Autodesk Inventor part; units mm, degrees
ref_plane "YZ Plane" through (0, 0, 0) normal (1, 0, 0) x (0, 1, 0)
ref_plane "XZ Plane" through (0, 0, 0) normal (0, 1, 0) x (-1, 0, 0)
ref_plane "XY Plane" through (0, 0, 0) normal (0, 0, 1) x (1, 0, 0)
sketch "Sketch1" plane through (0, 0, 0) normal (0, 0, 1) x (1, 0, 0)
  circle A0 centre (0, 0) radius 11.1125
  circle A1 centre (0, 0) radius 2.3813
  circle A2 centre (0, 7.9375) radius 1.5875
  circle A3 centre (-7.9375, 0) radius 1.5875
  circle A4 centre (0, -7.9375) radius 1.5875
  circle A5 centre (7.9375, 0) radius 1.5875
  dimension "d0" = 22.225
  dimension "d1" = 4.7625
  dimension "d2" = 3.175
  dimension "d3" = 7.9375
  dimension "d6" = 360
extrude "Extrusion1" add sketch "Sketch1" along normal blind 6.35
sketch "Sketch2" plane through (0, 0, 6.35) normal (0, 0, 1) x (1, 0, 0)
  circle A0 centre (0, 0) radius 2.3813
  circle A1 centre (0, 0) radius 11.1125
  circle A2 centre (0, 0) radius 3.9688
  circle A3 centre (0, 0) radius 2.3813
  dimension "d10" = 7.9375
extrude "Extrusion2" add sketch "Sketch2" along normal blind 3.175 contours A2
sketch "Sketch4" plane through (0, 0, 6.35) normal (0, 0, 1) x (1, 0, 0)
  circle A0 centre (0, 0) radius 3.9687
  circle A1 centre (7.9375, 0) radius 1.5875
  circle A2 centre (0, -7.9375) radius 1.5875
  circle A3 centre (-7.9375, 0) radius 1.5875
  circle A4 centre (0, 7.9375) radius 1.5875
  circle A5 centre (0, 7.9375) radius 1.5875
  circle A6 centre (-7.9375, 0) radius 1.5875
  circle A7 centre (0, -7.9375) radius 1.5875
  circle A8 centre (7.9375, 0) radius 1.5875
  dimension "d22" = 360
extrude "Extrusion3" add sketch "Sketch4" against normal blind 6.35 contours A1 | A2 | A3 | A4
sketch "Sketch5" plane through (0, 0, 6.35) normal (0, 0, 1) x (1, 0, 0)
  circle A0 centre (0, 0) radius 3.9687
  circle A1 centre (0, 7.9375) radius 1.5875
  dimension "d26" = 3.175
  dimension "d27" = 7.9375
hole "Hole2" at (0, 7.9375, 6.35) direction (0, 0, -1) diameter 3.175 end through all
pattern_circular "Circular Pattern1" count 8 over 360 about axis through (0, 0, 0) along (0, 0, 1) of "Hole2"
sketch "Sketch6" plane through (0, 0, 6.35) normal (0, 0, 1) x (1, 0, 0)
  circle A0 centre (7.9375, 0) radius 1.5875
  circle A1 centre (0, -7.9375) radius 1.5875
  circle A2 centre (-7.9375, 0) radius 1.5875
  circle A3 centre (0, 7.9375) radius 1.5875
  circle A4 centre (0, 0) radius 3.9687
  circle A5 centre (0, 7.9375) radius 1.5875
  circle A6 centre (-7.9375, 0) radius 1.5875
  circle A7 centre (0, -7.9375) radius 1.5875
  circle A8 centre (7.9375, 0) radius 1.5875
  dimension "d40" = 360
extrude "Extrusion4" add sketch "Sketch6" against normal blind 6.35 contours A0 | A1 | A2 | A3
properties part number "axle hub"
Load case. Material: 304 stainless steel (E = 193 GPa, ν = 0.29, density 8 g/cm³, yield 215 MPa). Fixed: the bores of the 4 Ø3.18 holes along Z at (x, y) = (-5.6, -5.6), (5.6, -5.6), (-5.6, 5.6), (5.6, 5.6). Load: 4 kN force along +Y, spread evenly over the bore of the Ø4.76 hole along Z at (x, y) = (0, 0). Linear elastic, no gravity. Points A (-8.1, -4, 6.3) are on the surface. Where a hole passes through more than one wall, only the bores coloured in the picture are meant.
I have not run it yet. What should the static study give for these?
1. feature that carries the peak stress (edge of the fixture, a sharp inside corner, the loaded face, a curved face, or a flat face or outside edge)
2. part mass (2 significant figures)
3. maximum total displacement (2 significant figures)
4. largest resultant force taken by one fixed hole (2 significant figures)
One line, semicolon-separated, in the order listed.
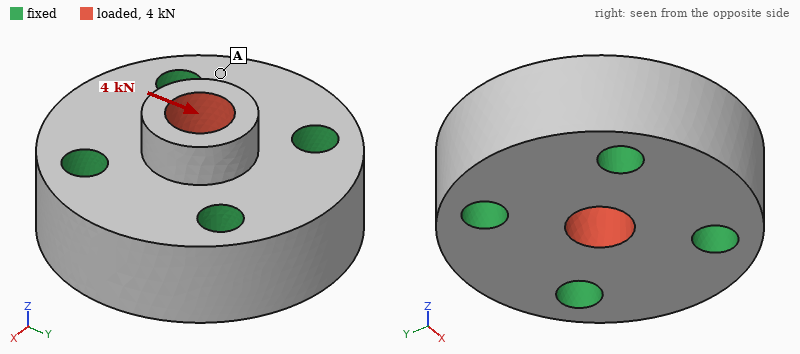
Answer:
the loaded face; 18 g; 4.3 µm; 1.1 kN
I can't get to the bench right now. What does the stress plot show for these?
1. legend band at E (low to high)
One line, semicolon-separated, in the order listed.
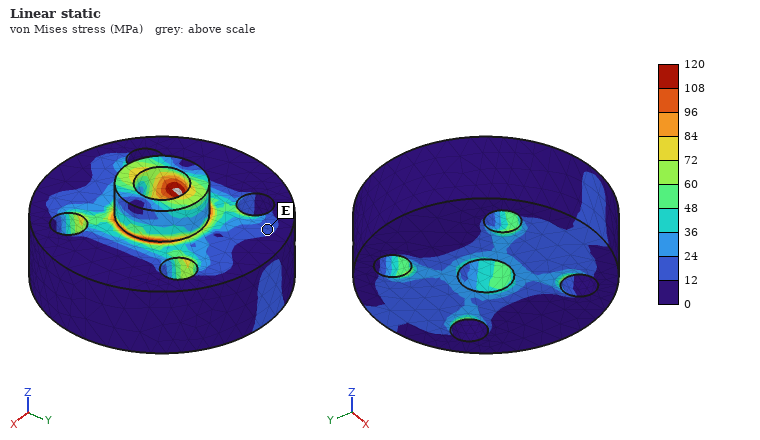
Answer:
12 to 24 MPa
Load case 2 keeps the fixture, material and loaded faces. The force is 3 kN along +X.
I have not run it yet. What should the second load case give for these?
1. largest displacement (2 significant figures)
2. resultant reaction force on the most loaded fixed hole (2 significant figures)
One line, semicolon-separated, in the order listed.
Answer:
3.3 µm; 810 N
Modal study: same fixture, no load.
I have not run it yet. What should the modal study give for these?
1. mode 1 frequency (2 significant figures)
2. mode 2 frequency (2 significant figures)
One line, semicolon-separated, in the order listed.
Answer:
110 kHz; 110 kHz
